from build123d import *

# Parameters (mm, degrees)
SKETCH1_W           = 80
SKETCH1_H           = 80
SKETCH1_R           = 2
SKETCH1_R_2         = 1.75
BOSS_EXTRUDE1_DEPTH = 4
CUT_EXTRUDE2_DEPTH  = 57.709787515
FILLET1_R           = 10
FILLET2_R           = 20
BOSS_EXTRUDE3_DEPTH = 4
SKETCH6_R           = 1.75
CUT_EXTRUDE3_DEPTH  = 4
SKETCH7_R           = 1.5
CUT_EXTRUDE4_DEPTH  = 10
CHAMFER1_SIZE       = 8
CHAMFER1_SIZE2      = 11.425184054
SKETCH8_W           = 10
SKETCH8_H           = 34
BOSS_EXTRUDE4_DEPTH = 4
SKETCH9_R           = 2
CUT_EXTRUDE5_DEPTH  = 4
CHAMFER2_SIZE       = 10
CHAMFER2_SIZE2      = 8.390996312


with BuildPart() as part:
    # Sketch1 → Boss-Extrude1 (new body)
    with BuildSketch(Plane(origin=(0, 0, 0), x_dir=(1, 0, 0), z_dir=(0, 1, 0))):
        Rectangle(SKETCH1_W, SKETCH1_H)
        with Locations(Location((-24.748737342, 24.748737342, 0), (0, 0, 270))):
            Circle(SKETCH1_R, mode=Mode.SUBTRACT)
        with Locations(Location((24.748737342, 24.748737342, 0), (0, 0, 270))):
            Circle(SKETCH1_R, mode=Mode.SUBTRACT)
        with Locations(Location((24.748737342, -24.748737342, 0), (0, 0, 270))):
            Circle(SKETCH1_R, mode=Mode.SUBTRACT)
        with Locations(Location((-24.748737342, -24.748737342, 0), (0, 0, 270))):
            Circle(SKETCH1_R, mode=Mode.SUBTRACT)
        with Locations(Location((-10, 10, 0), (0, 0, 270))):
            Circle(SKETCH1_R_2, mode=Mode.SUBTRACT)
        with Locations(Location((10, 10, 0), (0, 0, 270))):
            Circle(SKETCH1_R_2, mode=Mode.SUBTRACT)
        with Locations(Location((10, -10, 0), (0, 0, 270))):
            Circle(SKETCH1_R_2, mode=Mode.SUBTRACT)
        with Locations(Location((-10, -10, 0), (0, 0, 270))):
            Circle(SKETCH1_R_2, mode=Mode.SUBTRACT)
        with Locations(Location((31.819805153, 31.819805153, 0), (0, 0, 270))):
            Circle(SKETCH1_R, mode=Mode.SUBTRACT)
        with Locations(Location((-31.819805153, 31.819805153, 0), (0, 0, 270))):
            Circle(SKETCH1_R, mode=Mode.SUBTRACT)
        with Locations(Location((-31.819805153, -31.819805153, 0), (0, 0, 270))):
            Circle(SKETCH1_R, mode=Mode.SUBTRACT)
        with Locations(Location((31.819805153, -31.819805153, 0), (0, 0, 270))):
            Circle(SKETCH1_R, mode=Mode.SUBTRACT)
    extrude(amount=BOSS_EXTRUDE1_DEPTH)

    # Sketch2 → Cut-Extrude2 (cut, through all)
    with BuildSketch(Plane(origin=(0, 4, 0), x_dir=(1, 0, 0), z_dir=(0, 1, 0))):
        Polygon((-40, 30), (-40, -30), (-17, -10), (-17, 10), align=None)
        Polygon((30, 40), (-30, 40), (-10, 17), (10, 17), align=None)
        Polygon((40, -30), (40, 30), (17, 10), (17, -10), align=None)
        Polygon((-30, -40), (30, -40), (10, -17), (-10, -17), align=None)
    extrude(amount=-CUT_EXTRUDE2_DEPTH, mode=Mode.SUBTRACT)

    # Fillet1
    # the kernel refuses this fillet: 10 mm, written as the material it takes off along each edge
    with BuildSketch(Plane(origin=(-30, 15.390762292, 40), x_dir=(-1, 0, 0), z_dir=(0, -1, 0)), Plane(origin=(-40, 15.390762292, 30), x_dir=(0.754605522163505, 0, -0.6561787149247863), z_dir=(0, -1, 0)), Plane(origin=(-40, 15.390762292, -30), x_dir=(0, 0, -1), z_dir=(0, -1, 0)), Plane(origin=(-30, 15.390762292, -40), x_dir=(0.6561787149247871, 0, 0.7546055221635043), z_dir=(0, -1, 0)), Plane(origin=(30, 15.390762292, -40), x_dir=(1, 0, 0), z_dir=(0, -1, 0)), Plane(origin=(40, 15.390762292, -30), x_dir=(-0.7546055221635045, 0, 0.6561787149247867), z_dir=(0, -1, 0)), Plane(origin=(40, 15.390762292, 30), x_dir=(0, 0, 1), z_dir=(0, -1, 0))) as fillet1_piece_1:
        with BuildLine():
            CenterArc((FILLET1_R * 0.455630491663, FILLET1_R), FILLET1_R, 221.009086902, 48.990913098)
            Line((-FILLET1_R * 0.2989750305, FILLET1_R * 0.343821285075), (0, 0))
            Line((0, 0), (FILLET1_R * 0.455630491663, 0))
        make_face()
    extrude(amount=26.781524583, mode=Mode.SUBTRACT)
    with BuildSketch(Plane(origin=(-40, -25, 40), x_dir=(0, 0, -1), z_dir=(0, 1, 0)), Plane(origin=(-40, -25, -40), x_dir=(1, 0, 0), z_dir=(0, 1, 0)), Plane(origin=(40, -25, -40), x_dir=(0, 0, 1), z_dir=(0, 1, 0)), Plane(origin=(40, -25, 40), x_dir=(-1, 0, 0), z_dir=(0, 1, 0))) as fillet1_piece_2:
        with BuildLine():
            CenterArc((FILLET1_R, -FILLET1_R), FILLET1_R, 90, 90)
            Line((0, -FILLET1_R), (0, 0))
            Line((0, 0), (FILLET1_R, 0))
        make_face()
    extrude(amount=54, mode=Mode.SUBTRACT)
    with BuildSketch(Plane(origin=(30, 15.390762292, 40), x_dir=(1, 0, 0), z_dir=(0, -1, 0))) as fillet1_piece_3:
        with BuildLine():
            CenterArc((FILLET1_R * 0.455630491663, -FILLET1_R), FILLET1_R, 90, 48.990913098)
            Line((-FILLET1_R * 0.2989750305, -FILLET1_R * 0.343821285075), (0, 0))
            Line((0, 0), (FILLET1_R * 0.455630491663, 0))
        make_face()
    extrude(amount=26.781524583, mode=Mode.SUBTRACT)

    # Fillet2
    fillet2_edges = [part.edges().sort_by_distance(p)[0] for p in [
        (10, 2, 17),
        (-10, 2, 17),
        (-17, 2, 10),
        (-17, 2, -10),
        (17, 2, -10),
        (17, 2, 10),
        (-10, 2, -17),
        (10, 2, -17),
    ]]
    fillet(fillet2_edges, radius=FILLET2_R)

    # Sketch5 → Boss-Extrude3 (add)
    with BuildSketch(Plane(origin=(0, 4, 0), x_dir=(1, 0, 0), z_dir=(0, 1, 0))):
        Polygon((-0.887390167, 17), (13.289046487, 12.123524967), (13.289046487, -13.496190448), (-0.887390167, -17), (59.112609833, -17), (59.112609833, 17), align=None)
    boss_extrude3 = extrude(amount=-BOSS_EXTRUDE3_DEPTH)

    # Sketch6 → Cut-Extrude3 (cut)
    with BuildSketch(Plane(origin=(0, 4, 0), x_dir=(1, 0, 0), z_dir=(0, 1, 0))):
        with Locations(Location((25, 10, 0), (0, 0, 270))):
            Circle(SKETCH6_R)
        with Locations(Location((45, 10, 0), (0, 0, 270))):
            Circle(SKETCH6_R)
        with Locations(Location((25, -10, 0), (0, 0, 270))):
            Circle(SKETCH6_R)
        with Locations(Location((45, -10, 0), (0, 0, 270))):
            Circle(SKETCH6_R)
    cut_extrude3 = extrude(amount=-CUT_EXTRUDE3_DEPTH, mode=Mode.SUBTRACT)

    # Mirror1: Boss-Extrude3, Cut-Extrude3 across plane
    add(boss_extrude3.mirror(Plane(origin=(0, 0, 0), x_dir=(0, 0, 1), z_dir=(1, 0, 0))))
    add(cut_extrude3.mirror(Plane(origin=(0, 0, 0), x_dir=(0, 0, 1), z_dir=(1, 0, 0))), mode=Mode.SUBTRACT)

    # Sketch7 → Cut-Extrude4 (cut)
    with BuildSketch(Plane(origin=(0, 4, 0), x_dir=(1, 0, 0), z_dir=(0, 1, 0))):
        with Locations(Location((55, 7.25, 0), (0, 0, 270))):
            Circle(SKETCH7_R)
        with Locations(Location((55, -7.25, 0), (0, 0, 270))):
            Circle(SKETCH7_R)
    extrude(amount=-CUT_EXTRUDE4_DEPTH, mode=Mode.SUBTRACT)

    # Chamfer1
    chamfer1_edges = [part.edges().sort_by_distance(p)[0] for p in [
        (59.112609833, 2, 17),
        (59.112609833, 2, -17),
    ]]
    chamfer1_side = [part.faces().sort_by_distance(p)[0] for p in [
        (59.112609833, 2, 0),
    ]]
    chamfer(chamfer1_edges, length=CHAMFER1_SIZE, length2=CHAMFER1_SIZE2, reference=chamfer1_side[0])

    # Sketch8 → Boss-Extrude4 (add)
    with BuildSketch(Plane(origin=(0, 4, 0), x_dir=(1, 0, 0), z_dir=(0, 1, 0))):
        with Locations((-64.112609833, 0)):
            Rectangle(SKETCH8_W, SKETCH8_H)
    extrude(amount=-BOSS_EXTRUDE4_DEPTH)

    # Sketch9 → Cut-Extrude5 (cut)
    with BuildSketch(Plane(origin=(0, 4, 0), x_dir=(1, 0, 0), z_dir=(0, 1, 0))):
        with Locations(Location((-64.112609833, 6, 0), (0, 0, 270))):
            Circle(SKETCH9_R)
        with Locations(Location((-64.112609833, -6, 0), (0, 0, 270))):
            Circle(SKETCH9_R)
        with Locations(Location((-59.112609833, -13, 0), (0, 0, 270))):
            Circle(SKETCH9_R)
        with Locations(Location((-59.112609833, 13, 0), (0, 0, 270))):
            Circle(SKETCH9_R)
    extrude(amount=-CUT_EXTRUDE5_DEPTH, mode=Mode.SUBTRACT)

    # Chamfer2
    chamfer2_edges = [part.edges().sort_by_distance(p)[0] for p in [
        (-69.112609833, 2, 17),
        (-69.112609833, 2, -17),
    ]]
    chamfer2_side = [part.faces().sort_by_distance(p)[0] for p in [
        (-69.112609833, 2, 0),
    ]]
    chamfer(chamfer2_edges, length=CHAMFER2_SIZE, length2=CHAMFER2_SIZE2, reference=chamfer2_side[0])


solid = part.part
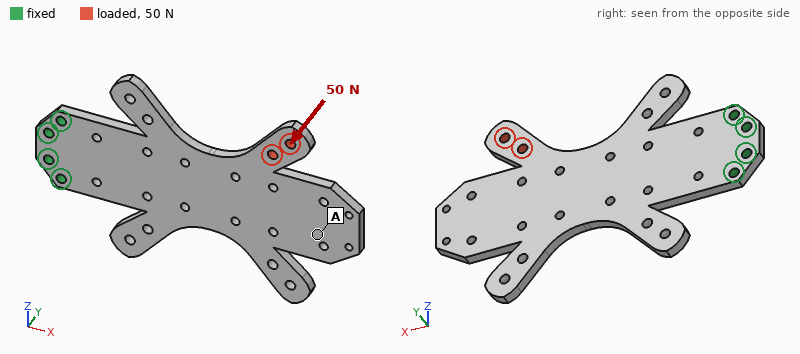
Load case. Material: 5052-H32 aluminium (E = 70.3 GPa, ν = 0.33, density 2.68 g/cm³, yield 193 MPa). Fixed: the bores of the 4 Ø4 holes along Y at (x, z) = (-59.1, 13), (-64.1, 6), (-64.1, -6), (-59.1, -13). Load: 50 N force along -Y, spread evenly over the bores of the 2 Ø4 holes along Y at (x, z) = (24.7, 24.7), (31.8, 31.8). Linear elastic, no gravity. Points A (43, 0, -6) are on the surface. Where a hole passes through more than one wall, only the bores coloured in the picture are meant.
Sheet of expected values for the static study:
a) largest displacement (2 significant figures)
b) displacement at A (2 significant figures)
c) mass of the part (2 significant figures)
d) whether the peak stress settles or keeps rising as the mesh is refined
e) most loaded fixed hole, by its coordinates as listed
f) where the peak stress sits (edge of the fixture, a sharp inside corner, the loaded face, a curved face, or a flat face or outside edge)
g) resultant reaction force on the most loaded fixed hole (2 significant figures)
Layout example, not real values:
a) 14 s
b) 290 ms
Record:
a) 1.4 mm
b) 1.1 mm
c) 57 g
d) keeps rising
e) (-59.1, 13)
f) edge of the fixture
g) 150 N
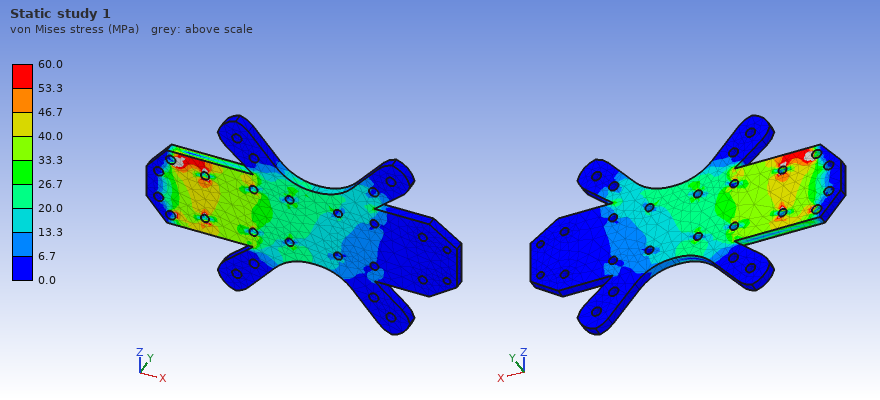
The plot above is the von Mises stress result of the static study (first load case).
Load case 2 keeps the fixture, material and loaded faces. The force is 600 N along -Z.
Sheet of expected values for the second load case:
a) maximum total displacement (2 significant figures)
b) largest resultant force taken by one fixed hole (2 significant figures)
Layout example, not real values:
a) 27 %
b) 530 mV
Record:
a) 0.25 mm
b) 1.8 kN
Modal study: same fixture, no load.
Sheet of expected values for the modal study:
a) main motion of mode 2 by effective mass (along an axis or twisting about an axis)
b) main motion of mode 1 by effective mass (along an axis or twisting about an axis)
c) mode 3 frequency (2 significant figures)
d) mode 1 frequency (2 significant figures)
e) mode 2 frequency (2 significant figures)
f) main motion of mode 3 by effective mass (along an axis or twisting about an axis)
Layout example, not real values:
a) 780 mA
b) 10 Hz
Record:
a) twisting about X
b) along Y
c) 1400 Hz
d) 220 Hz
e) 870 Hz
f) along Y
